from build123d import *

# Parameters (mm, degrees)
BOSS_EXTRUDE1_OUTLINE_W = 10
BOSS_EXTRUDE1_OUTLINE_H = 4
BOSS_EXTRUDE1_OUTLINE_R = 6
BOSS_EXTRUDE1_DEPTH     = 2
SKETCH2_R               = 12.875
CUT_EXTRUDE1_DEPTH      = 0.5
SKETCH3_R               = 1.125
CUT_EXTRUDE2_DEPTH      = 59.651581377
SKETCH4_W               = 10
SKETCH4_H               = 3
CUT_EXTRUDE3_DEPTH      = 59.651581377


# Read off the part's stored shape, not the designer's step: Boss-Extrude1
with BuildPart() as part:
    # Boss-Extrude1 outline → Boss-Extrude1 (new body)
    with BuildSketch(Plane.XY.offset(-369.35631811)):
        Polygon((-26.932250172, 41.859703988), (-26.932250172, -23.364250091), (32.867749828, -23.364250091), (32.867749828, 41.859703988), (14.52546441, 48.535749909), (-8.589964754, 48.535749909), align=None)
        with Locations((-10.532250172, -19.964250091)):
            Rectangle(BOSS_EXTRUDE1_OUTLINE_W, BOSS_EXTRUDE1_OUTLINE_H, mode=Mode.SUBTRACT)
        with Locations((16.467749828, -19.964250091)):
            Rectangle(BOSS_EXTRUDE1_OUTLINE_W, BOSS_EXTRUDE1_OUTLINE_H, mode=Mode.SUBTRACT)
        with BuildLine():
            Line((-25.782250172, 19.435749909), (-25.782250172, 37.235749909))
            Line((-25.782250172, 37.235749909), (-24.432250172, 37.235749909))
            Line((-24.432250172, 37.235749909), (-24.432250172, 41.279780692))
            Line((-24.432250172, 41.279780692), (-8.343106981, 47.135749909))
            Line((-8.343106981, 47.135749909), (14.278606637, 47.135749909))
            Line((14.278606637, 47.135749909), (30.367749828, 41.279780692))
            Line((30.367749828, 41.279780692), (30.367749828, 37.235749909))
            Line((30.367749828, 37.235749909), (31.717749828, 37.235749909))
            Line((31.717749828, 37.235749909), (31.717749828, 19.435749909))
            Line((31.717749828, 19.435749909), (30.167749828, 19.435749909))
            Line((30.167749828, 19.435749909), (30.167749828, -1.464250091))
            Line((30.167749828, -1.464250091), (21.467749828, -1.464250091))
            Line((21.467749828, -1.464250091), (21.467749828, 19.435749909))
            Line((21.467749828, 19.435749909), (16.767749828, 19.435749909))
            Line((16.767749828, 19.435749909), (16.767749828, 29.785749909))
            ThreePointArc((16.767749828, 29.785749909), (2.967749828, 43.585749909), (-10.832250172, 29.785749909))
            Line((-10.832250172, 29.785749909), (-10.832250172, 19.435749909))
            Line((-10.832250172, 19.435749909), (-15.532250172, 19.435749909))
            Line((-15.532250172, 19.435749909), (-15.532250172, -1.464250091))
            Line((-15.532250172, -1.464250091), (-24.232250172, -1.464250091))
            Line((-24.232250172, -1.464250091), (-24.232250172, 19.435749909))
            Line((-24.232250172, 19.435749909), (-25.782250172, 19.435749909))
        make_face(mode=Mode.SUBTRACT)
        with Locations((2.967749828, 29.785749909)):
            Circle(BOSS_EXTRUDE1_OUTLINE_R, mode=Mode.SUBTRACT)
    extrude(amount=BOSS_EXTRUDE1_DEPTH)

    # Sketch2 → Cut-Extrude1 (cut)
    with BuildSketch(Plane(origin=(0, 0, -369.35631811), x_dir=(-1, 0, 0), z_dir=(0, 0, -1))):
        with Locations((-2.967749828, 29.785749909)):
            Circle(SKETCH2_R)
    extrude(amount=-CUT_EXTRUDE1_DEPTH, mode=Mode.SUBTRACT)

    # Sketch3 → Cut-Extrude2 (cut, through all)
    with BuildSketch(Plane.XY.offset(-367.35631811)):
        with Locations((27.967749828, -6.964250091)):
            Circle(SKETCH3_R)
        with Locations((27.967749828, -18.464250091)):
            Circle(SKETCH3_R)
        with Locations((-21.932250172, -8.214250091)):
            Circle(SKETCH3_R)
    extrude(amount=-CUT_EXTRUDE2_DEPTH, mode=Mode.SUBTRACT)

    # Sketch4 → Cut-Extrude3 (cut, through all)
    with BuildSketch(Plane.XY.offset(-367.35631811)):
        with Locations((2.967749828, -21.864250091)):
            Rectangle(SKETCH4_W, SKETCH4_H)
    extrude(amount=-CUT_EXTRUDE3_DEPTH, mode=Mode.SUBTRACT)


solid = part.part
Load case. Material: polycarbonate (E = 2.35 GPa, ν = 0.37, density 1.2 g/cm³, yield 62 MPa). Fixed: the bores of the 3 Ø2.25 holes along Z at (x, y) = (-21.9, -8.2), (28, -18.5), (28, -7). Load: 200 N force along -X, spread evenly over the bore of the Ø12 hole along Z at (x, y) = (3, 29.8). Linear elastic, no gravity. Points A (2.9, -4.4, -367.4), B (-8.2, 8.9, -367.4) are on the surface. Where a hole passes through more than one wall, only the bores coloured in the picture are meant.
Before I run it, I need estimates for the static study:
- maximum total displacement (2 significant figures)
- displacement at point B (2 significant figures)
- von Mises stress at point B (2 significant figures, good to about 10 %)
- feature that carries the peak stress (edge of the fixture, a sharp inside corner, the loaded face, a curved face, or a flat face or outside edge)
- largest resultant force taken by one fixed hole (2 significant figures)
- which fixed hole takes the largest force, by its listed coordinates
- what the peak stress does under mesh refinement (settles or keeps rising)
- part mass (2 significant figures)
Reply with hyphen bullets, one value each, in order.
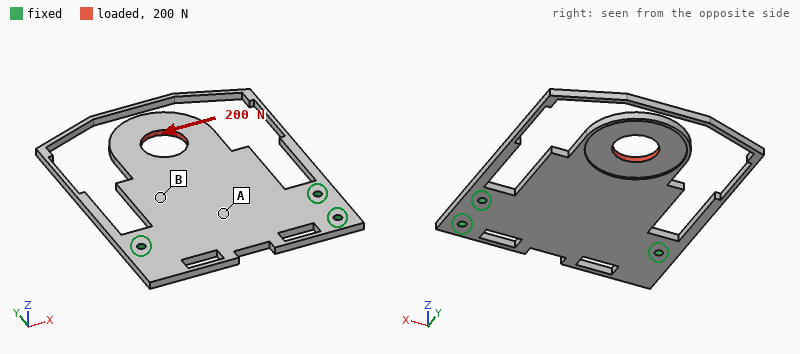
- 0.67 mm
- 0.17 mm
- 8.6 MPa
- edge of the fixture
- 180 N
- (-21.9, -8.2)
- keeps rising
- 6.2 g
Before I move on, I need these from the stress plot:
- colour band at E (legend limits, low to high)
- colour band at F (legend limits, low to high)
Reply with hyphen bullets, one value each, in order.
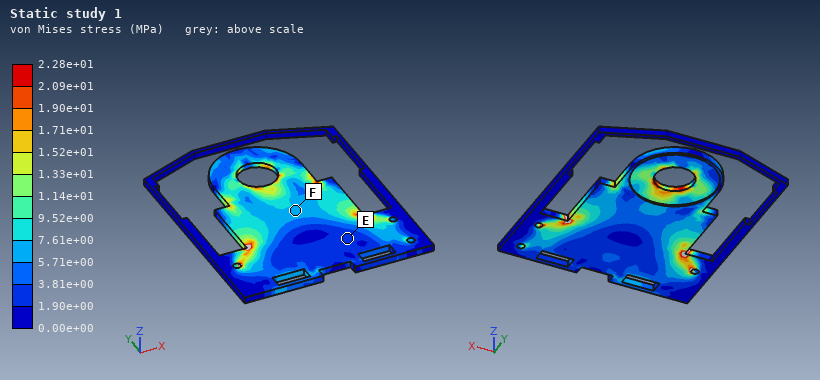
- 1.90e+00 to 3.81e+00 MPa
- 5.71e+00 to 7.61e+00 MPa
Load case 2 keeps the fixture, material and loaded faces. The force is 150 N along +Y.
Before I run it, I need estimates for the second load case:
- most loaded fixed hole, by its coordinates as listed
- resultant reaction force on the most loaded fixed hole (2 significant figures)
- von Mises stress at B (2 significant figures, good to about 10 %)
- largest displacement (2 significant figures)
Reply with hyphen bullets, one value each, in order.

- (-21.9, -8.2)
- 69 N
- 3.9 MPa
- 0.96 mm
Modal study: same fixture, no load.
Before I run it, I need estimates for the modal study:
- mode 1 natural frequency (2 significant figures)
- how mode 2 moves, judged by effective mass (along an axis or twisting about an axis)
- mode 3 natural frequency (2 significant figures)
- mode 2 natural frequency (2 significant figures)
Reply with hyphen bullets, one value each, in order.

- 120 Hz
- along Z
- 210 Hz
- 200 Hz
